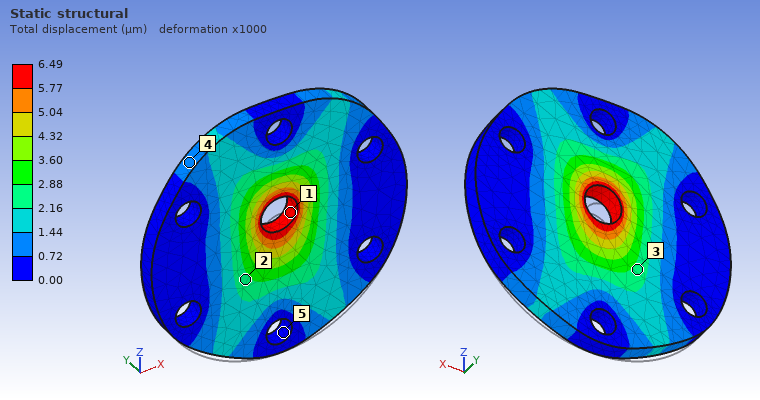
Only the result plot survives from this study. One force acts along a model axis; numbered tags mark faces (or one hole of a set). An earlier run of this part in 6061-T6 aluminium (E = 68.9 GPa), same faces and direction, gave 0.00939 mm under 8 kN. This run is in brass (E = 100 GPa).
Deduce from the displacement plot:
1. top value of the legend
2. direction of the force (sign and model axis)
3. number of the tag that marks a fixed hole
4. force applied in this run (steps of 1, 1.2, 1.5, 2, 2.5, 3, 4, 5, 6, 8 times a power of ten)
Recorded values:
6.49 µm
+Z
5
8 kN
